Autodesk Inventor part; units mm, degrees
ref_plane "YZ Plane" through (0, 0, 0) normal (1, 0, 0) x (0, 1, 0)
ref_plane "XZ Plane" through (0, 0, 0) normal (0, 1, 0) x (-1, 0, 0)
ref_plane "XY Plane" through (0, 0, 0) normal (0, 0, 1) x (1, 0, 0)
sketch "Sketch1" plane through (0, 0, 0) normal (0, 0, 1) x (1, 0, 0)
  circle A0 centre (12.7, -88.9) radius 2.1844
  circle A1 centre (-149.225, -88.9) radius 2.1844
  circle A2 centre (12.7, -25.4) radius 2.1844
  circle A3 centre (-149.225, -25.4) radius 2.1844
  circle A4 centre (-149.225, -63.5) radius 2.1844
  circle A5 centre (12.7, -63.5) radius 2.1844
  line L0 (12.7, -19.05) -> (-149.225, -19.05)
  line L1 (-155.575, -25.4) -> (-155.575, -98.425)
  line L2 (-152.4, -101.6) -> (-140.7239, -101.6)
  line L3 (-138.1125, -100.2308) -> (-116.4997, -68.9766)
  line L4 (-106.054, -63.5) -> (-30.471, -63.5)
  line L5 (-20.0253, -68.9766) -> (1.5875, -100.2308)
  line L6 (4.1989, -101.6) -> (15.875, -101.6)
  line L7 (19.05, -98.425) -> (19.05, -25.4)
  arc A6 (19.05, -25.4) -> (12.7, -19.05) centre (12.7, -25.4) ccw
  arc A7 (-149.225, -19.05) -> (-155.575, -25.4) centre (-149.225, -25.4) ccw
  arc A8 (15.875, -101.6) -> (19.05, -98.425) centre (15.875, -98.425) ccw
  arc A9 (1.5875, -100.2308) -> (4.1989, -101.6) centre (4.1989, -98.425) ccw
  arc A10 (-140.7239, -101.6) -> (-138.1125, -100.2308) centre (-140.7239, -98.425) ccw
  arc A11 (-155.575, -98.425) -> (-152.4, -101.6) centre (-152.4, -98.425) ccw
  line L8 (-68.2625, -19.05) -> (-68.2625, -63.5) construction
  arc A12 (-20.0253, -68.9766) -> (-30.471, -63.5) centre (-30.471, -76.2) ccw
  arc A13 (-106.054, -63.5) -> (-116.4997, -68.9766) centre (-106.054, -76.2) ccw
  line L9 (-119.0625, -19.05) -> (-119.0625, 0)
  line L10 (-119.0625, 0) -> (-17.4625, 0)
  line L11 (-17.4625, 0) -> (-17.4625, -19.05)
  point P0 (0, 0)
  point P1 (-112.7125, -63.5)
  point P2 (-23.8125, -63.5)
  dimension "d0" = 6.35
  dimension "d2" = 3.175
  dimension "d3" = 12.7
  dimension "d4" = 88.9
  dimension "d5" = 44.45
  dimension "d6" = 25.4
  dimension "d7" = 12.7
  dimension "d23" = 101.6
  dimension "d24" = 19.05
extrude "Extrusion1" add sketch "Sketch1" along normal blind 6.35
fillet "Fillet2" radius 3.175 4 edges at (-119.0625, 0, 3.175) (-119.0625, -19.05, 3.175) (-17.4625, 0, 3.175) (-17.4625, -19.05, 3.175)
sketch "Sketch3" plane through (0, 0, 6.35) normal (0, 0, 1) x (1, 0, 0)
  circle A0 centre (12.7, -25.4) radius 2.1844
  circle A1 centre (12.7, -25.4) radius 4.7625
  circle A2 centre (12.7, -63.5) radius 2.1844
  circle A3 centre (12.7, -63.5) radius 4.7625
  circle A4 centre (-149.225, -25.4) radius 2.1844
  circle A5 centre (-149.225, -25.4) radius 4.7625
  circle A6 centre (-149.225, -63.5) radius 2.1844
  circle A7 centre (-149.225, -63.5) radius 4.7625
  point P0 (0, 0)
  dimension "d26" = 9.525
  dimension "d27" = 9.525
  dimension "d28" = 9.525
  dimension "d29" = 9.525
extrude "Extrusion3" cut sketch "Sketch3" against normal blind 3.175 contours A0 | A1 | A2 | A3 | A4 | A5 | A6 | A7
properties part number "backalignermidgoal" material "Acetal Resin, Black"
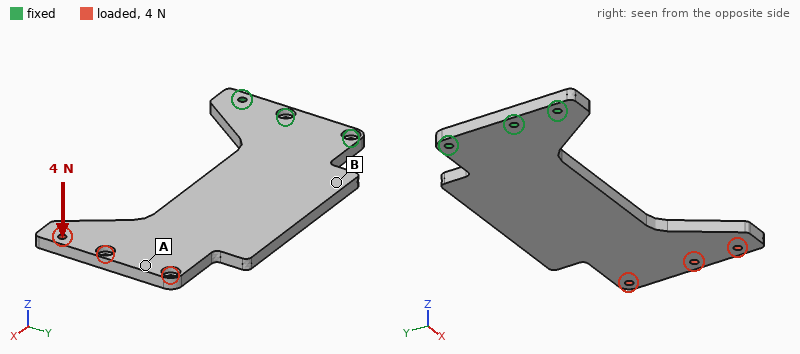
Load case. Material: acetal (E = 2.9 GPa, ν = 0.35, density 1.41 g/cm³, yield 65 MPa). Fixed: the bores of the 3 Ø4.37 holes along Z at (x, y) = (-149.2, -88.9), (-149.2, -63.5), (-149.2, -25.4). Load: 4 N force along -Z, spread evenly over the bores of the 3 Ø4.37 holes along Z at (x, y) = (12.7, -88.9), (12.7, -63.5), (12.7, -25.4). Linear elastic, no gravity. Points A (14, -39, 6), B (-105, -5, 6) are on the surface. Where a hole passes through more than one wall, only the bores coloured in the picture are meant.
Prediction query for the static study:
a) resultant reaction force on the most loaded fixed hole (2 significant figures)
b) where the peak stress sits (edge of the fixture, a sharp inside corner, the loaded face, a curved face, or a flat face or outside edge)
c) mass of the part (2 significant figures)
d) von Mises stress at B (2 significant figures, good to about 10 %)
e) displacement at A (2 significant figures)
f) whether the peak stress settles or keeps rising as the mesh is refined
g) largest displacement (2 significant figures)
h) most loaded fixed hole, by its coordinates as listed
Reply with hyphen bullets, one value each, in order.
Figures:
- 14 N
- edge of the fixture
- 110 g
- 0.60 MPa
- 1.9 mm
- keeps rising
- 2.1 mm
- (-149.2, -63.5)
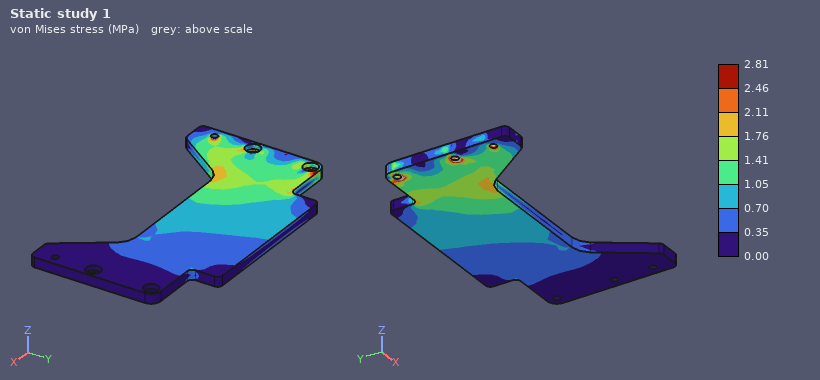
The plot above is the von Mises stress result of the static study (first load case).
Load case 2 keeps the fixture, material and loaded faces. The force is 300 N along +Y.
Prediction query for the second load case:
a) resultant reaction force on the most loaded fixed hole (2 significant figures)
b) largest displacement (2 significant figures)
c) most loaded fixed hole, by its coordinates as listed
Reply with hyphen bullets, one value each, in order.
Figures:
- 890 N
- 2.3 mm
- (-149.2, -25.4)
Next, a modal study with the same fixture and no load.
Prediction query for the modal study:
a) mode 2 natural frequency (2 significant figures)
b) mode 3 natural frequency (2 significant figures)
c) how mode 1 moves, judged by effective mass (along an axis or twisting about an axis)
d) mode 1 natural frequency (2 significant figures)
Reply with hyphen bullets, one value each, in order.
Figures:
- 170 Hz
- 340 Hz
- along Z
- 42 Hz
